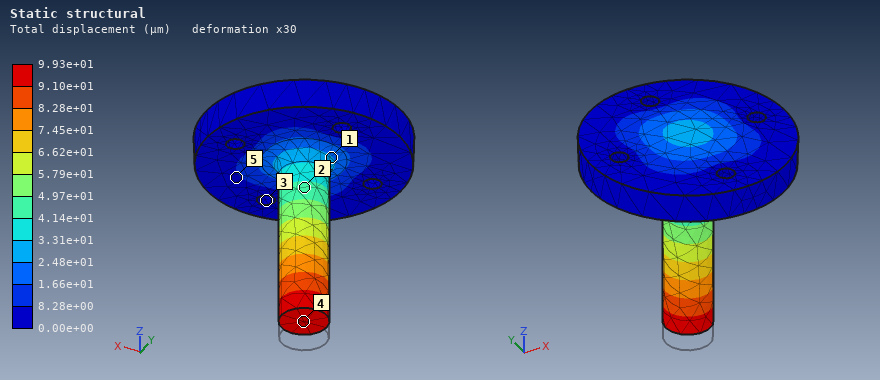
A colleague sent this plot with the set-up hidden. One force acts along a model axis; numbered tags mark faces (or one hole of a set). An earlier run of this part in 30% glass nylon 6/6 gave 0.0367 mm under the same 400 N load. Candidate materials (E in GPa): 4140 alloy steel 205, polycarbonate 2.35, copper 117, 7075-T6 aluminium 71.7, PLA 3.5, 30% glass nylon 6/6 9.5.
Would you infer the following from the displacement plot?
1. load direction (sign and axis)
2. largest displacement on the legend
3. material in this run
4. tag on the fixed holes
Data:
+Z
9.93e+01 µm
PLA
3
